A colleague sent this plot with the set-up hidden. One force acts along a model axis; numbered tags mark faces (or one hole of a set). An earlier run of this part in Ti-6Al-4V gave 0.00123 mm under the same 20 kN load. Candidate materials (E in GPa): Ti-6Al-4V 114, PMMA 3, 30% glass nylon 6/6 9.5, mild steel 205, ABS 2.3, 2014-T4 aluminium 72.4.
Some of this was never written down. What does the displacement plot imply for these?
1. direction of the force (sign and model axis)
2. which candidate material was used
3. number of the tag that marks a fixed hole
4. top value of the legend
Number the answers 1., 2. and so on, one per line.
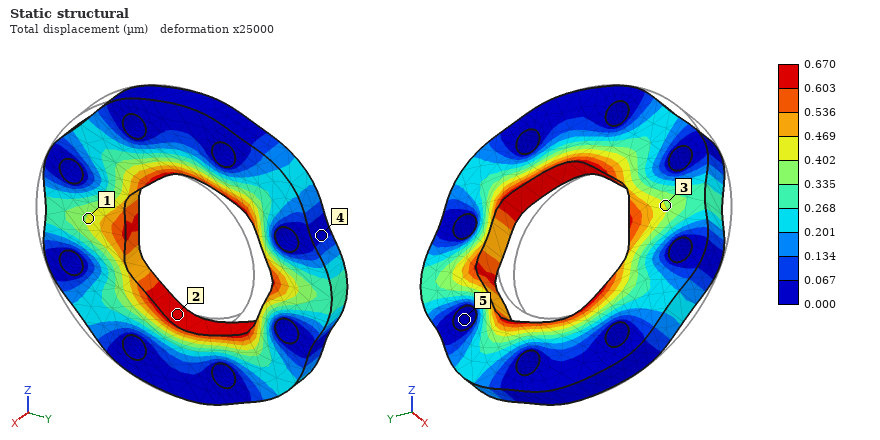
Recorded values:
1. +Y
2. mild steel
3. 5
4. 0.670 µm
